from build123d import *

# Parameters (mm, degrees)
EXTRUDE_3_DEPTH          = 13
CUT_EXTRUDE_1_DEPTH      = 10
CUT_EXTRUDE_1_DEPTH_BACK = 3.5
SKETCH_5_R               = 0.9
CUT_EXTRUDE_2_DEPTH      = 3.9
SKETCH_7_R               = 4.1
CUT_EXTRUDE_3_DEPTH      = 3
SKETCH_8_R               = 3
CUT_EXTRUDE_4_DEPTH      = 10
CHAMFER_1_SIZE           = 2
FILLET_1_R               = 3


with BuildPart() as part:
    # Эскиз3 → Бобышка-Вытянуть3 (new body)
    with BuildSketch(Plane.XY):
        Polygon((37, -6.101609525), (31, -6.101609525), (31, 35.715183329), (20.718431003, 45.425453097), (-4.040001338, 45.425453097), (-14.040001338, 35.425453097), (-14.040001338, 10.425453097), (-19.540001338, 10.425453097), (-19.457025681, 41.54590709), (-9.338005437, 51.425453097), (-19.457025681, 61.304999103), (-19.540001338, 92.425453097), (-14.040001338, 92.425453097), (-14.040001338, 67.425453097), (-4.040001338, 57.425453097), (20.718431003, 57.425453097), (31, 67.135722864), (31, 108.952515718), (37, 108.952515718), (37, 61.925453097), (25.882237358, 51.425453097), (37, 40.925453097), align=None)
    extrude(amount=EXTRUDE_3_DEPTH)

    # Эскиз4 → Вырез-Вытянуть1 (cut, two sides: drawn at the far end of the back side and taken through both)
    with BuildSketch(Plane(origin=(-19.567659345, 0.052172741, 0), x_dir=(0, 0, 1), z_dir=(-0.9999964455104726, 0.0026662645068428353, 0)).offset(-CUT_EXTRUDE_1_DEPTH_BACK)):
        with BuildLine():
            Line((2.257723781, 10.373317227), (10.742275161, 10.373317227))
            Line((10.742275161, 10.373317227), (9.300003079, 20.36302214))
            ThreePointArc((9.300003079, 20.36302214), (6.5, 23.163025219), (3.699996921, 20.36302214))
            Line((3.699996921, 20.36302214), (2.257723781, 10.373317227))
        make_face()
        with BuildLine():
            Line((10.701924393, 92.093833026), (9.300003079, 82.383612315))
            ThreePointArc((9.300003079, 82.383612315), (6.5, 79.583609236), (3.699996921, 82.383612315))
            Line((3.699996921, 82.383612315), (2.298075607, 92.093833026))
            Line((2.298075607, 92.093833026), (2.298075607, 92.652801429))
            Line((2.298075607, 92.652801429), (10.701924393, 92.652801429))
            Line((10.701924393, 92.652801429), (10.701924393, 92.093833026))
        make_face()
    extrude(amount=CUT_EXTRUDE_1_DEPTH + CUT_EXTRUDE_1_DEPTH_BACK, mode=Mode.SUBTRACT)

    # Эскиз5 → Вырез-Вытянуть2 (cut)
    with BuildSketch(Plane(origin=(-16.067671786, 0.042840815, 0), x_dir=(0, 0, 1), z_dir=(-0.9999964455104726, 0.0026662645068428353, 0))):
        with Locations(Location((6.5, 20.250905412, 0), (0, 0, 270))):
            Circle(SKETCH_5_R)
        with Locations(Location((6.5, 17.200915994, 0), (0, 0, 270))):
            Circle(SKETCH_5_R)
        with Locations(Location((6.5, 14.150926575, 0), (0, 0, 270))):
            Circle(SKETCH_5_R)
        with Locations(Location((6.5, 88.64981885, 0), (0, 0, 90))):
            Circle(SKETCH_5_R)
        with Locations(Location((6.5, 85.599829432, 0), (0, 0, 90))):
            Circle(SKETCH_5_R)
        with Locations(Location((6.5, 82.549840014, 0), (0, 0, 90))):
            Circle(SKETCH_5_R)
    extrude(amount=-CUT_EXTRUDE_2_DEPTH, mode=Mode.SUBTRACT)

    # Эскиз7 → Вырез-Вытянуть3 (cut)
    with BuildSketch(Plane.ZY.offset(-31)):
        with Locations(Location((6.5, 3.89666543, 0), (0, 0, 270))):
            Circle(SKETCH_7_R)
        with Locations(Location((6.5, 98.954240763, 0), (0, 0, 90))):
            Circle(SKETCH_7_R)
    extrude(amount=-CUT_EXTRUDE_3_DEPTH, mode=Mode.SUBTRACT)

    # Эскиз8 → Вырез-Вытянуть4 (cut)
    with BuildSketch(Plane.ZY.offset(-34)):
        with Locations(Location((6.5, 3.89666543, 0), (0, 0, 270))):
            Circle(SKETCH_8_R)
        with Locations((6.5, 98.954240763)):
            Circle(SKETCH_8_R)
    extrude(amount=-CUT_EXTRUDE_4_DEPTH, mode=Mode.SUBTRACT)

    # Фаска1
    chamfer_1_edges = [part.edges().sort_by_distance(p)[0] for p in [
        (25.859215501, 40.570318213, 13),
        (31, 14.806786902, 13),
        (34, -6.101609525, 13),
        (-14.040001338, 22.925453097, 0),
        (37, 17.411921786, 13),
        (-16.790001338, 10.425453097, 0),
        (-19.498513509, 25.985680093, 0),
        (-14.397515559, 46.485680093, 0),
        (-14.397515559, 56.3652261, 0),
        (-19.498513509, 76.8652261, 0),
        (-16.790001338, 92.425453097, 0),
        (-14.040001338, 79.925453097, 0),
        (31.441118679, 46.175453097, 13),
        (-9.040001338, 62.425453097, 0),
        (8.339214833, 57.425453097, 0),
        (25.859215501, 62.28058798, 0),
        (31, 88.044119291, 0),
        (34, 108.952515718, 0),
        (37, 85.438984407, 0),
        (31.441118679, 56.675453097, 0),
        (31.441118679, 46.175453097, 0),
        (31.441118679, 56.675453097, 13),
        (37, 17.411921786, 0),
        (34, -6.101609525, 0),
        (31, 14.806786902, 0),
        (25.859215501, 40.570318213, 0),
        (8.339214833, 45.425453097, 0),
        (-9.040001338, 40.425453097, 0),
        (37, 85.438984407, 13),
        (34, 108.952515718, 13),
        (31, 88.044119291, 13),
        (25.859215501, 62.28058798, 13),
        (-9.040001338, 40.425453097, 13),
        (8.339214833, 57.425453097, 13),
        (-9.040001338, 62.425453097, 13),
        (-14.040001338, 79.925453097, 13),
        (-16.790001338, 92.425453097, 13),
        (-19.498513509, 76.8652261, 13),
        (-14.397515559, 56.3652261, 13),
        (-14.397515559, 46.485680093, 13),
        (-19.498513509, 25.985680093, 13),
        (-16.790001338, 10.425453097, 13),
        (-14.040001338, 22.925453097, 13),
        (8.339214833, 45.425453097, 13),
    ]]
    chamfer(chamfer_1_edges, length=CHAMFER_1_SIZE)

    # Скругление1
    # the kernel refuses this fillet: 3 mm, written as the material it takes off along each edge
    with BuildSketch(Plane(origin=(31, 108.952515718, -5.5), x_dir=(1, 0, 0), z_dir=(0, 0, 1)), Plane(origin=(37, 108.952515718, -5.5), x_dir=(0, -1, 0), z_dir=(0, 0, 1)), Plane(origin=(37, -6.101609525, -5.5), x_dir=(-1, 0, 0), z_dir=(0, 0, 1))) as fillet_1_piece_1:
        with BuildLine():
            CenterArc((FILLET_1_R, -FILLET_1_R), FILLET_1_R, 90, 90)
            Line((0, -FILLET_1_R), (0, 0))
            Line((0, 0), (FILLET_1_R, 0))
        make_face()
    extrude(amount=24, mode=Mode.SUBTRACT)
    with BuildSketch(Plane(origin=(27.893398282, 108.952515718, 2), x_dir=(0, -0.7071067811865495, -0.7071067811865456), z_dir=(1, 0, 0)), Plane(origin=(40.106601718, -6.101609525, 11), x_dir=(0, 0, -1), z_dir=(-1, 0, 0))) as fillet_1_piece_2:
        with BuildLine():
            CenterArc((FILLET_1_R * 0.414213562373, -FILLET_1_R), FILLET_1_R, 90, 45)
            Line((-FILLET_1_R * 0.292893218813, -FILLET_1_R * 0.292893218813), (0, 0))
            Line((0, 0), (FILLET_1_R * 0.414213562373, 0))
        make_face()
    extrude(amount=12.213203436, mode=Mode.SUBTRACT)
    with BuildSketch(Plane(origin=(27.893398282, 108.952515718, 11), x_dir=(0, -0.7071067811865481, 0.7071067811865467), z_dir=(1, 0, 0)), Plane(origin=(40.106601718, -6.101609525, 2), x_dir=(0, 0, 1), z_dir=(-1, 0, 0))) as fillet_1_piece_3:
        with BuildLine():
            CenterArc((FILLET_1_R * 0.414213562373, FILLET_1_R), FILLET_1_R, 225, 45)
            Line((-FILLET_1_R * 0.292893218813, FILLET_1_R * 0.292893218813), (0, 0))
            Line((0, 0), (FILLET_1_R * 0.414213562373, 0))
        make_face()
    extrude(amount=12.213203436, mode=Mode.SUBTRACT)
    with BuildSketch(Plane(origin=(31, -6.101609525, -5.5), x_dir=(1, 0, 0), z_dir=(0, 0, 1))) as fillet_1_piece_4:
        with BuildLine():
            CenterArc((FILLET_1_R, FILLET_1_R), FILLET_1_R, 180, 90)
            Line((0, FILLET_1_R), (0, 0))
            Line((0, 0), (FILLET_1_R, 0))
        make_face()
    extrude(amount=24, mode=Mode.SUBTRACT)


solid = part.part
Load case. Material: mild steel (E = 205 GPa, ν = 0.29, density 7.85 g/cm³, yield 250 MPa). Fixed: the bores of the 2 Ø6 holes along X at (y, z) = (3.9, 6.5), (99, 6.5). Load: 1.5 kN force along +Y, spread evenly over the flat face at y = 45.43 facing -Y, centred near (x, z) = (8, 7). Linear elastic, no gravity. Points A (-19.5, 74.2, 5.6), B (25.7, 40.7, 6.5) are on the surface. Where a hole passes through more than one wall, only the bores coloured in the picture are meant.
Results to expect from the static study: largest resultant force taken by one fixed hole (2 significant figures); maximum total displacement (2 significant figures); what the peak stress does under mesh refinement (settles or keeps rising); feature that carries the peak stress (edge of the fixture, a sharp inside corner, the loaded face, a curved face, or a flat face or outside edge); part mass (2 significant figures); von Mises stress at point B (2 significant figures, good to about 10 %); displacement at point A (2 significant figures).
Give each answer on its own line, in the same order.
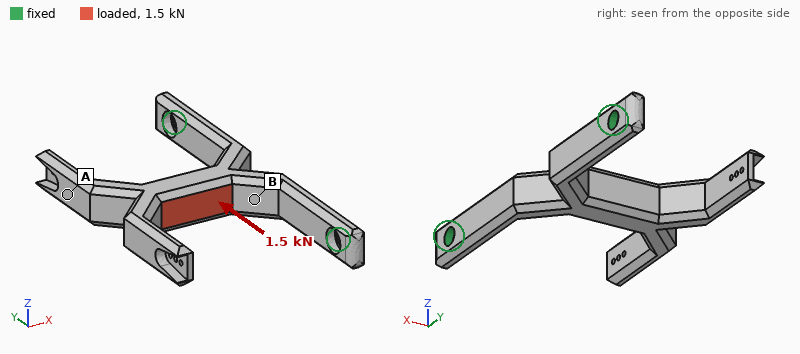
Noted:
940 N
0.23 mm
keeps rising
edge of the fixture
150 g
100 MPa
0.19 mm
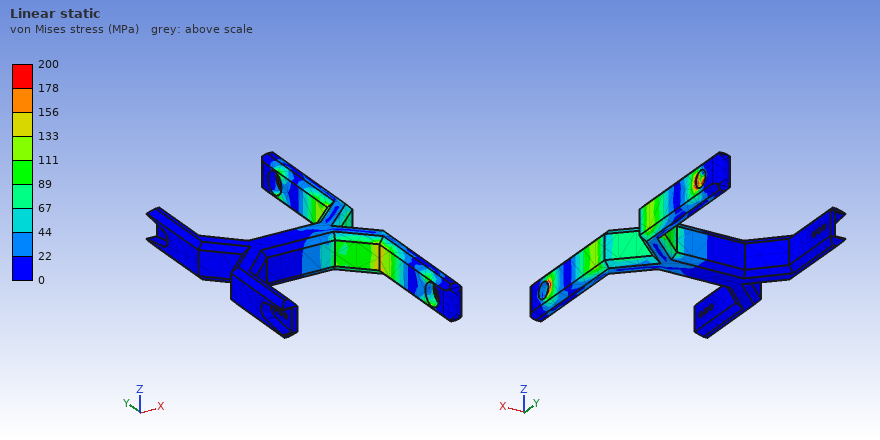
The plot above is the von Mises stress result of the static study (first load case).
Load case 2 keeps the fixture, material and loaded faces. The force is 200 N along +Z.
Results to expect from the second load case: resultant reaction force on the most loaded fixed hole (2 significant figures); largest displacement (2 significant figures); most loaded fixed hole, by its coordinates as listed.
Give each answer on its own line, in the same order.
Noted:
120 N
0.13 mm
(3.9, 6.5)
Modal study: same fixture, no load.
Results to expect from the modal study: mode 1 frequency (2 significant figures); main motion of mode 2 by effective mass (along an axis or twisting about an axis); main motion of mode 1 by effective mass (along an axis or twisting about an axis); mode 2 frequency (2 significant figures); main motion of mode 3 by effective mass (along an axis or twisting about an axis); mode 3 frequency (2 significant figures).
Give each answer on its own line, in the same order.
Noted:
640 Hz
along Y
along Z
1300 Hz
along X
1900 Hz
